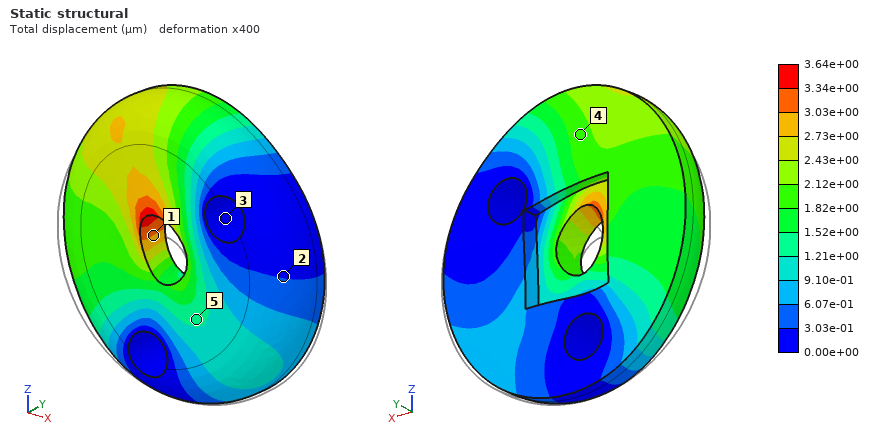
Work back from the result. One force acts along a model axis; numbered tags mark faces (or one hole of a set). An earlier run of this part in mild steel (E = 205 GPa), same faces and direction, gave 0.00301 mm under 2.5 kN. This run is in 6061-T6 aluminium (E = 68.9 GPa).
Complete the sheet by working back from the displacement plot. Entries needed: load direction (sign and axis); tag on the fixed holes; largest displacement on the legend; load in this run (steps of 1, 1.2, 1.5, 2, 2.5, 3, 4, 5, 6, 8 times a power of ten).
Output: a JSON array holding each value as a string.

["+Z", "3", "3.64e+00 µm", "1 kN"]
